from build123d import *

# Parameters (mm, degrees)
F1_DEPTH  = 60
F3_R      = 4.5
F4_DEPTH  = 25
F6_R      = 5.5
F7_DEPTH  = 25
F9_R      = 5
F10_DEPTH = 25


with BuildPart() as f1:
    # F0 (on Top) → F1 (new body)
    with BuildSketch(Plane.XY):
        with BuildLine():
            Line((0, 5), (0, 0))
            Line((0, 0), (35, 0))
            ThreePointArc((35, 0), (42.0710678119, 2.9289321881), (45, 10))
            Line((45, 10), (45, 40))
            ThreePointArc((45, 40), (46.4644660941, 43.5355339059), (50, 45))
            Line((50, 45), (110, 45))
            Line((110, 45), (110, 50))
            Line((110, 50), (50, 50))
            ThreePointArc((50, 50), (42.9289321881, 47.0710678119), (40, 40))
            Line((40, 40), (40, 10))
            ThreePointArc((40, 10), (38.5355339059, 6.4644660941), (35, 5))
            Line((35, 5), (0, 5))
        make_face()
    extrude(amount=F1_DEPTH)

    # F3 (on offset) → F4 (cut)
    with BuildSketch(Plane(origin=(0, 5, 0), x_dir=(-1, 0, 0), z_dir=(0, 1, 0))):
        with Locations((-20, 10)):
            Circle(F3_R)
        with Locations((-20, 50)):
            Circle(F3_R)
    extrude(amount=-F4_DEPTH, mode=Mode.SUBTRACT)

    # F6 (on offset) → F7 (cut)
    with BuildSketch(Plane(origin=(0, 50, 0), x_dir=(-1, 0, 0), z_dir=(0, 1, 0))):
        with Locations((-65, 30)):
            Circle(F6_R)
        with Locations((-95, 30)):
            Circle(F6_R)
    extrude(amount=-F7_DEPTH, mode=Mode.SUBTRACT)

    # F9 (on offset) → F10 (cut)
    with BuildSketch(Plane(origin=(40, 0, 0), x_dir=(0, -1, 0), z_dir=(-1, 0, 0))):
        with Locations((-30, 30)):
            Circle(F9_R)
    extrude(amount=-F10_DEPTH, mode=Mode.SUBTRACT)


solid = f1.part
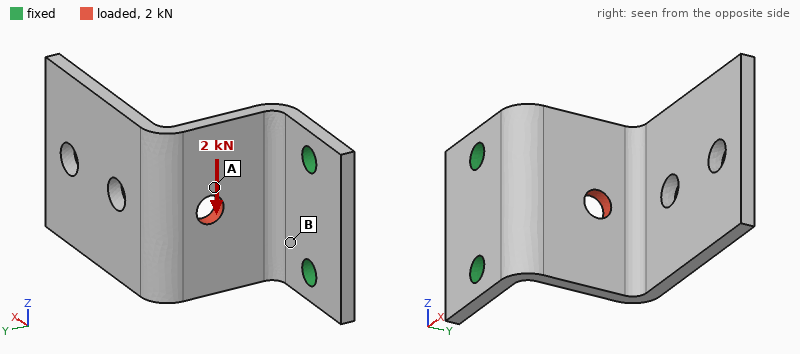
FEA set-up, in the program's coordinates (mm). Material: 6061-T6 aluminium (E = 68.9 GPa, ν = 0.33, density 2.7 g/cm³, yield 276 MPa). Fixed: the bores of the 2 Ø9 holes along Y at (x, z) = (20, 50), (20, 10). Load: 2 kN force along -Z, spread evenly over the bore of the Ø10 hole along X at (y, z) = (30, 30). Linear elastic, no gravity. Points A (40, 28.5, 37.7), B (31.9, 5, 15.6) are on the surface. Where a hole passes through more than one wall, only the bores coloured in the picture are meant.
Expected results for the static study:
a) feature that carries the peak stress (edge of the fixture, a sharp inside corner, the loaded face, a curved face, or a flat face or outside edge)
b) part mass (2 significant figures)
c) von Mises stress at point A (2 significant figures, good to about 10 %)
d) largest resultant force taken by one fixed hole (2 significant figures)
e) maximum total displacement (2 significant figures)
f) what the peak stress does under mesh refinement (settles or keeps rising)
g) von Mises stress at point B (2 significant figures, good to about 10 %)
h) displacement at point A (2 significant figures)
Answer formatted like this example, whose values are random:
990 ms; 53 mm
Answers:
edge of the fixture; 110 g; 28 MPa; 1.9 kN; 0.27 mm; keeps rising; 76 MPa; 0.14 mm
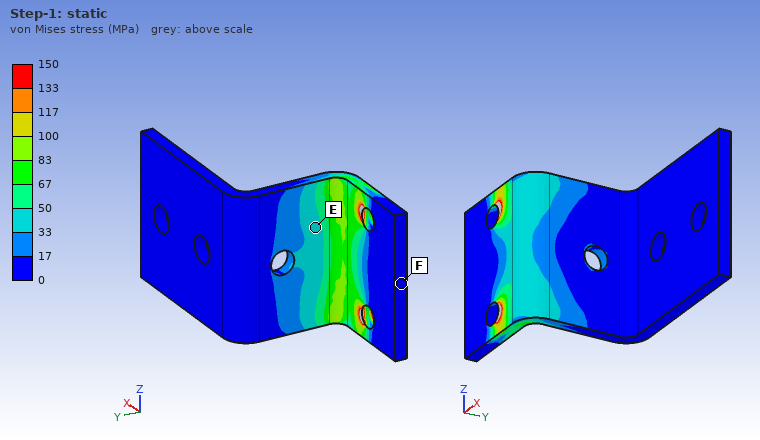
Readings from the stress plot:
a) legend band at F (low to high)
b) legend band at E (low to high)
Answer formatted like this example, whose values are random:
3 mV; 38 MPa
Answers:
0 to 17 MPa; 33 to 50 MPa
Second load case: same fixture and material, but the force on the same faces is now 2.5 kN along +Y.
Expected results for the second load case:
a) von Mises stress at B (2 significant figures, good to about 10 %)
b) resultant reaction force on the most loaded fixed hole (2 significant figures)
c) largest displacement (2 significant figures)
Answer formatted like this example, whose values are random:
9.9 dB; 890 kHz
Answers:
97 MPa; 1.3 kN; 1.1 mm
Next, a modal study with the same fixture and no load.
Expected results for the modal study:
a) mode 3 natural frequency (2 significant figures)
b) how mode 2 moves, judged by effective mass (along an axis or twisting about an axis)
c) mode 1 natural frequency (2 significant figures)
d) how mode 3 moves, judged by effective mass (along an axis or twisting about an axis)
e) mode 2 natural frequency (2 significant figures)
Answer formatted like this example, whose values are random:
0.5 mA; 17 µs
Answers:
1100 Hz; along Z; 340 Hz; along X; 760 Hz
